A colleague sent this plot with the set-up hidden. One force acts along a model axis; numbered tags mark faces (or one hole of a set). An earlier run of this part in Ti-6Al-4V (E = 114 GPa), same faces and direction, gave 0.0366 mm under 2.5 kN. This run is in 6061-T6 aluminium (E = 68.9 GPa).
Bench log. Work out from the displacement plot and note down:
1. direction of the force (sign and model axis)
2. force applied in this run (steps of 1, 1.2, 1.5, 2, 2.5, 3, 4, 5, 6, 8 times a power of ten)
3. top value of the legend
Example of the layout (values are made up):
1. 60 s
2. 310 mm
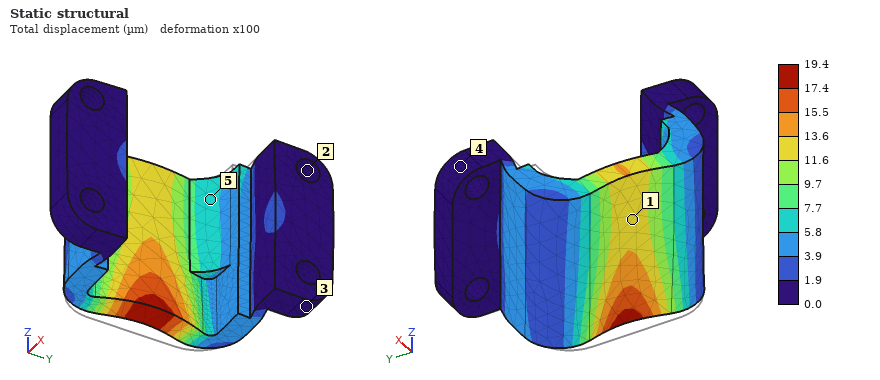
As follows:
1. +X
2. 800 N
3. 19.4 µm
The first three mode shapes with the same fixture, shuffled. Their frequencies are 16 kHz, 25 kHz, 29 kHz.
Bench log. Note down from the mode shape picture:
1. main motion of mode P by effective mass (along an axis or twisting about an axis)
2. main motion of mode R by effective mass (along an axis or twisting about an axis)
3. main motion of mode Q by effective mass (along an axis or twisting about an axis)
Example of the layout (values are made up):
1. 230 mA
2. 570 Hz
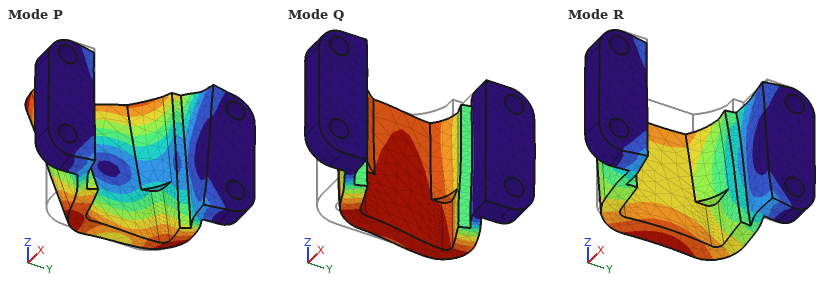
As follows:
1. twisting about X
2. along Z
3. along Y
